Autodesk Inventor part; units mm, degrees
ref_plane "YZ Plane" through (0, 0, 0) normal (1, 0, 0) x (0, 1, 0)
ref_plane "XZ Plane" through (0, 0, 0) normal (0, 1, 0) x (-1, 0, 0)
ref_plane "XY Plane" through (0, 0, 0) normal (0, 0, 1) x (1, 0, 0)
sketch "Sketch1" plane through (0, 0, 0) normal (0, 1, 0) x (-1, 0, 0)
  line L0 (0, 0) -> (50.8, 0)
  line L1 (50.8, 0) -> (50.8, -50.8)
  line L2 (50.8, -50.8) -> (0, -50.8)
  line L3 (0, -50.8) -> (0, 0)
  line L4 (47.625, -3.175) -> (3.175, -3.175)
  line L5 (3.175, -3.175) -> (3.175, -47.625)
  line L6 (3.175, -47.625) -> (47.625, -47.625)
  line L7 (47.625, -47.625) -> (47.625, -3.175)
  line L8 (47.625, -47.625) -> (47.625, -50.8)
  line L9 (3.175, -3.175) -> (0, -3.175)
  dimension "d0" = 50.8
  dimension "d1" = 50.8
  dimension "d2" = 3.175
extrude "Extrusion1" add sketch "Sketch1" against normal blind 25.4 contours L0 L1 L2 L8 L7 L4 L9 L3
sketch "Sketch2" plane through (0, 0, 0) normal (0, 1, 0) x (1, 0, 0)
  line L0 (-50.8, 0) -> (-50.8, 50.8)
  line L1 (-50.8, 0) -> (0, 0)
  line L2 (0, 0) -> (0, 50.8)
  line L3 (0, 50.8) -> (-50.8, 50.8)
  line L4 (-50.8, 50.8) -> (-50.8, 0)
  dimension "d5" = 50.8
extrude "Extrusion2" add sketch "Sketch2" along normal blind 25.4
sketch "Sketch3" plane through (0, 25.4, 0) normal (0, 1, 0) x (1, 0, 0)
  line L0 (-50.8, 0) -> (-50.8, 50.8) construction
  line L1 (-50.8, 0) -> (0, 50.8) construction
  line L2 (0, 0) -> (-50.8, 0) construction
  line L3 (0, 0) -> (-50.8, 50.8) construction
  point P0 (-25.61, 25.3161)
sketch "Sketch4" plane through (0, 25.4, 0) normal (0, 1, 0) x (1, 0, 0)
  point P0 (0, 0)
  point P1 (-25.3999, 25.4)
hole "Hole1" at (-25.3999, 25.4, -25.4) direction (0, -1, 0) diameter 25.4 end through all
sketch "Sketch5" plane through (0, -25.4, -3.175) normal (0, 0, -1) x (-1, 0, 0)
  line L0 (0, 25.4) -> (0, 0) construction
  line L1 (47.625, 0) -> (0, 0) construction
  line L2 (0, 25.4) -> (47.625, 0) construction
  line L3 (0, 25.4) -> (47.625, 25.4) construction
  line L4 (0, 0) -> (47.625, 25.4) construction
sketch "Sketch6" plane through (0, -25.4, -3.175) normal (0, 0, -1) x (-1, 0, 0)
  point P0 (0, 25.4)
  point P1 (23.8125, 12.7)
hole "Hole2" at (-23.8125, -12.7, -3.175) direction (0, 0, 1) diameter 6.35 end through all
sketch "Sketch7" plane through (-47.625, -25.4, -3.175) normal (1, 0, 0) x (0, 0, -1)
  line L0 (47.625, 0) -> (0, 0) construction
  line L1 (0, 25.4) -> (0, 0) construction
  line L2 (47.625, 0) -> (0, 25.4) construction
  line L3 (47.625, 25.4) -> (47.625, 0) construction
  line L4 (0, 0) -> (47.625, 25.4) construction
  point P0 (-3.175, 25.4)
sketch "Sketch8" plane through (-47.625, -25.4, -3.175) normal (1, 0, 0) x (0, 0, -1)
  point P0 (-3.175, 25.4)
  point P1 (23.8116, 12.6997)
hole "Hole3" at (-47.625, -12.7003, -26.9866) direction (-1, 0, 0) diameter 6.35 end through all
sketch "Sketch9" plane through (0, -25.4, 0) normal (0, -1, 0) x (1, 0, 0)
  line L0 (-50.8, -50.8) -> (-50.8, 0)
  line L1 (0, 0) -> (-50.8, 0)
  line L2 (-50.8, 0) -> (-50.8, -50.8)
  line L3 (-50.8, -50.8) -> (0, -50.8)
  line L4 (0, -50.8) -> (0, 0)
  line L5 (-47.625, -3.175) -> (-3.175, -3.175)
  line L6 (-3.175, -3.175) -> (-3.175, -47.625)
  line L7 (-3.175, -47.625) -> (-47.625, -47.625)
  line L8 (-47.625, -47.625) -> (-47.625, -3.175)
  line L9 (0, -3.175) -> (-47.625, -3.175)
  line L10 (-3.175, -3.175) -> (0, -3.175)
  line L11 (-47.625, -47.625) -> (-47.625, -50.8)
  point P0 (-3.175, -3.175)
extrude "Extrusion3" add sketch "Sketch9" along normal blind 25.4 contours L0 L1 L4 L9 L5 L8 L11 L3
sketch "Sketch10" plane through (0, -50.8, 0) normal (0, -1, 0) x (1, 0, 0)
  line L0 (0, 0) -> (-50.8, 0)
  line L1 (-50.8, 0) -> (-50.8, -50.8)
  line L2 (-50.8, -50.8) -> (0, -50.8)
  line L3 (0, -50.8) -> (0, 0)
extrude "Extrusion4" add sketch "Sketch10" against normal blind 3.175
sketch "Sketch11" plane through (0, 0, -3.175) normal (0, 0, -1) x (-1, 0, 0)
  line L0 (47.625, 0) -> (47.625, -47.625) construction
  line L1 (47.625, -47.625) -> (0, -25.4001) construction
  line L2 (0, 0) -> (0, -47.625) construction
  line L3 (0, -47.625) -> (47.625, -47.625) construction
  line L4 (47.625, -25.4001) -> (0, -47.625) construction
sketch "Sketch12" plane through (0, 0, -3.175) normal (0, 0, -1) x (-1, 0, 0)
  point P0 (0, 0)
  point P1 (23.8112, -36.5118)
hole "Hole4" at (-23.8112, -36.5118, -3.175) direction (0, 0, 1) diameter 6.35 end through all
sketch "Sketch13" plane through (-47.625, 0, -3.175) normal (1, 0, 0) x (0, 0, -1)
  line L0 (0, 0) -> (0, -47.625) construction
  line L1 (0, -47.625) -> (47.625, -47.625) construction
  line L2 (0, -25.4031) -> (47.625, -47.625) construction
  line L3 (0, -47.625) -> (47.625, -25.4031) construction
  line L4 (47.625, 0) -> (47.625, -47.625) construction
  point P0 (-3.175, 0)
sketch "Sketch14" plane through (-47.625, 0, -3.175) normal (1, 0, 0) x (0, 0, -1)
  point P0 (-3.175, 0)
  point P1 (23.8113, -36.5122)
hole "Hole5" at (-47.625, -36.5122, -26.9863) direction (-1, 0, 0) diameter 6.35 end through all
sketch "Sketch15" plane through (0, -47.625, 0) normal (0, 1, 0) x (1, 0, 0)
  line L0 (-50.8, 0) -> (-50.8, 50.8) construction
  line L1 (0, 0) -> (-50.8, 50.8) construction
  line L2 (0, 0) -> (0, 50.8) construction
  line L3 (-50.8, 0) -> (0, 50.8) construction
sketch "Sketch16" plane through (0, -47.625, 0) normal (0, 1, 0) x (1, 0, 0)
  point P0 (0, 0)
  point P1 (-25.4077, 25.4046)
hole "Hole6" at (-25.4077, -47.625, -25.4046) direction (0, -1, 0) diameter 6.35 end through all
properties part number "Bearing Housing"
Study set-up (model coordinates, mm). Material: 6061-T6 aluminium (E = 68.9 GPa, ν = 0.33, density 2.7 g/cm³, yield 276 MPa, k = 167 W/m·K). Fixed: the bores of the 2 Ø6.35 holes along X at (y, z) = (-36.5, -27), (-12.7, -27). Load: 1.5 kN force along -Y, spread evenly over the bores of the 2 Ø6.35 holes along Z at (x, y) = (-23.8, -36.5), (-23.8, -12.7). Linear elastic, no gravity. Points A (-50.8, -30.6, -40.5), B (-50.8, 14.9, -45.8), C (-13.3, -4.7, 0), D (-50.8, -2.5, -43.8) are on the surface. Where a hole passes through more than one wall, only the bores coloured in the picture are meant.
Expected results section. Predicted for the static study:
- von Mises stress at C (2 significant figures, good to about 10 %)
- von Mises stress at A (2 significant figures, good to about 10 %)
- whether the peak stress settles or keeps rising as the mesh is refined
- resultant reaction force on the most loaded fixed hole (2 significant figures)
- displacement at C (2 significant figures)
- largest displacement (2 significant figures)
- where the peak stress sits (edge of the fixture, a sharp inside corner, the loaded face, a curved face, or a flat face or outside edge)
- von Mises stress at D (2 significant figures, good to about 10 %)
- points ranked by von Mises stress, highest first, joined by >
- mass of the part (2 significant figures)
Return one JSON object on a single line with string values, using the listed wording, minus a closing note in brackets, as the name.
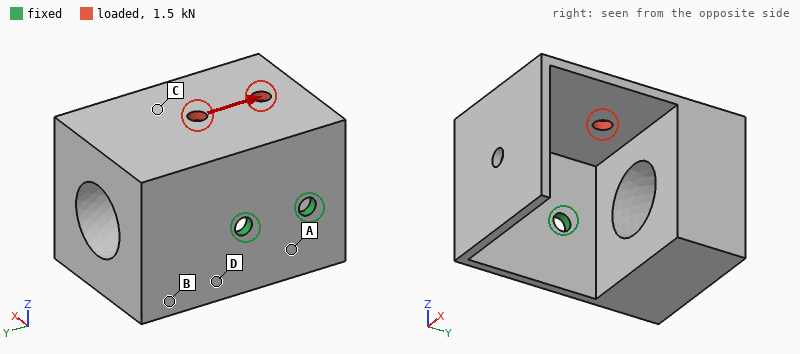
{"von Mises stress at C": "64 MPa", "von Mises stress at A": "32 MPa", "whether the peak stress settles or keeps rising as the mesh is refined": "keeps rising", "resultant reaction force on the most loaded fixed hole": "1.8 kN", "displacement at C": "0.43 mm", "largest displacement": "0.71 mm", "where the peak stress sits": "edge of the fixture", "von Mises stress at D": "93 MPa", "points ranked by von Mises stress, highest first, joined by >": "D > C > A > B", "mass of the part": "200 g"}
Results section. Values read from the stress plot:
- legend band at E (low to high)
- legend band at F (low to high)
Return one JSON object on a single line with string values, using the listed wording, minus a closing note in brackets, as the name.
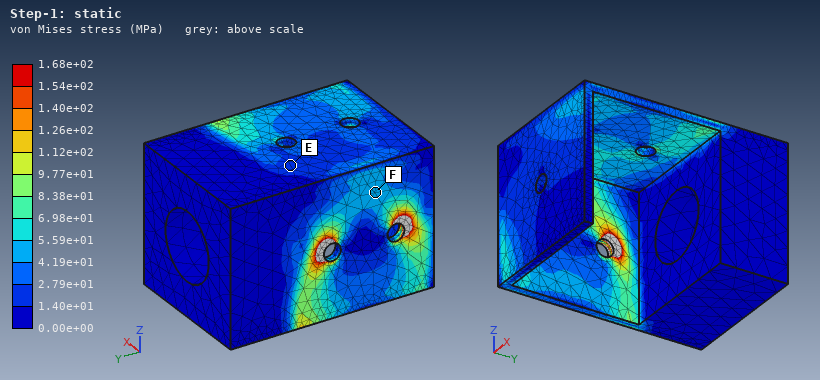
{"legend band at E": "1.40e+01 to 2.79e+01 MPa", "legend band at F": "4.19e+01 to 5.59e+01 MPa"}
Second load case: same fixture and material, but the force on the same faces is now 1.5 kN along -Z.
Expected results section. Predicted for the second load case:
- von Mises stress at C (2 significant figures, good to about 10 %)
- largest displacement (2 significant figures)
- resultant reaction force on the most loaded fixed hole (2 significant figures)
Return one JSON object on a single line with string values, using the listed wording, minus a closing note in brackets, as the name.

{"von Mises stress at C": "51 MPa", "largest displacement": "0.79 mm", "resultant reaction force on the most loaded fixed hole": "780 N"}
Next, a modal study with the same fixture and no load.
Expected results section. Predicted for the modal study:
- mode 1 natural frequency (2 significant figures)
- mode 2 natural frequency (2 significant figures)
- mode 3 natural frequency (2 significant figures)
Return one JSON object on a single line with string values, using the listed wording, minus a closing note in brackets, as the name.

{"mode 1 natural frequency": "510 Hz", "mode 2 natural frequency": "710 Hz", "mode 3 natural frequency": "1700 Hz"}
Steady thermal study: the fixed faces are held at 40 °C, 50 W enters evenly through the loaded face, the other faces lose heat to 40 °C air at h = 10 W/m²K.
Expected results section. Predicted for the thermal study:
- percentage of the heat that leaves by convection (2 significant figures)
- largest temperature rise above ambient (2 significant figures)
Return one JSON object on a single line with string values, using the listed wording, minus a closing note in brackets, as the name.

{"percentage of the heat that leaves by convection": "11 %", "largest temperature rise above ambient": "49 K"}
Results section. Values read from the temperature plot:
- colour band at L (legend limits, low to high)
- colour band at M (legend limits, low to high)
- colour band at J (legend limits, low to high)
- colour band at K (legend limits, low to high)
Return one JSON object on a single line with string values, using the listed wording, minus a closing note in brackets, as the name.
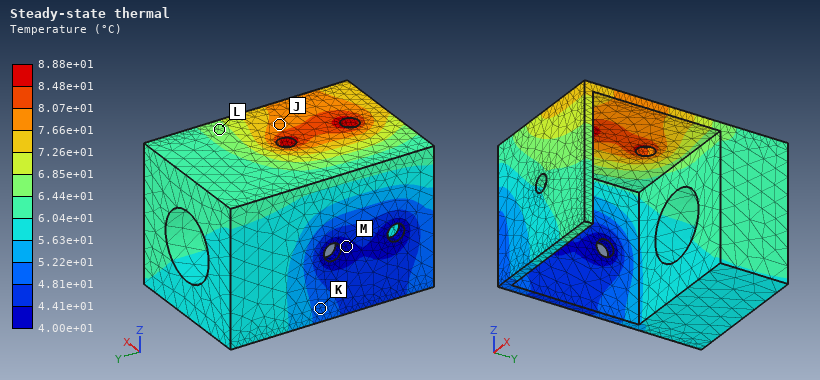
{"colour band at L": "6.44e+01 to 6.85e+01 °C", "colour band at M": "4.00e+01 to 4.41e+01 °C", "colour band at J": "7.66e+01 to 8.07e+01 °C", "colour band at K": "4.81e+01 to 5.22e+01 °C"}
